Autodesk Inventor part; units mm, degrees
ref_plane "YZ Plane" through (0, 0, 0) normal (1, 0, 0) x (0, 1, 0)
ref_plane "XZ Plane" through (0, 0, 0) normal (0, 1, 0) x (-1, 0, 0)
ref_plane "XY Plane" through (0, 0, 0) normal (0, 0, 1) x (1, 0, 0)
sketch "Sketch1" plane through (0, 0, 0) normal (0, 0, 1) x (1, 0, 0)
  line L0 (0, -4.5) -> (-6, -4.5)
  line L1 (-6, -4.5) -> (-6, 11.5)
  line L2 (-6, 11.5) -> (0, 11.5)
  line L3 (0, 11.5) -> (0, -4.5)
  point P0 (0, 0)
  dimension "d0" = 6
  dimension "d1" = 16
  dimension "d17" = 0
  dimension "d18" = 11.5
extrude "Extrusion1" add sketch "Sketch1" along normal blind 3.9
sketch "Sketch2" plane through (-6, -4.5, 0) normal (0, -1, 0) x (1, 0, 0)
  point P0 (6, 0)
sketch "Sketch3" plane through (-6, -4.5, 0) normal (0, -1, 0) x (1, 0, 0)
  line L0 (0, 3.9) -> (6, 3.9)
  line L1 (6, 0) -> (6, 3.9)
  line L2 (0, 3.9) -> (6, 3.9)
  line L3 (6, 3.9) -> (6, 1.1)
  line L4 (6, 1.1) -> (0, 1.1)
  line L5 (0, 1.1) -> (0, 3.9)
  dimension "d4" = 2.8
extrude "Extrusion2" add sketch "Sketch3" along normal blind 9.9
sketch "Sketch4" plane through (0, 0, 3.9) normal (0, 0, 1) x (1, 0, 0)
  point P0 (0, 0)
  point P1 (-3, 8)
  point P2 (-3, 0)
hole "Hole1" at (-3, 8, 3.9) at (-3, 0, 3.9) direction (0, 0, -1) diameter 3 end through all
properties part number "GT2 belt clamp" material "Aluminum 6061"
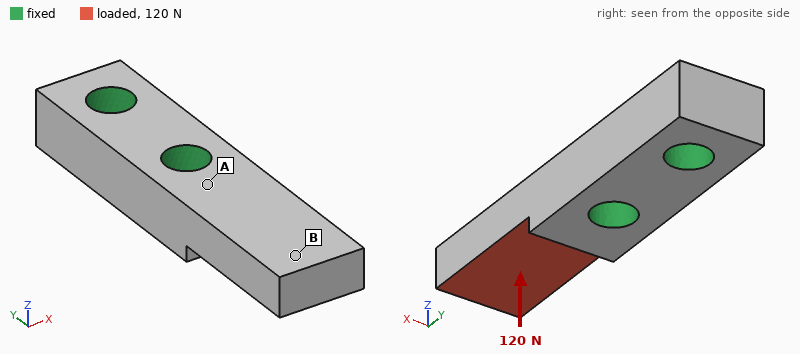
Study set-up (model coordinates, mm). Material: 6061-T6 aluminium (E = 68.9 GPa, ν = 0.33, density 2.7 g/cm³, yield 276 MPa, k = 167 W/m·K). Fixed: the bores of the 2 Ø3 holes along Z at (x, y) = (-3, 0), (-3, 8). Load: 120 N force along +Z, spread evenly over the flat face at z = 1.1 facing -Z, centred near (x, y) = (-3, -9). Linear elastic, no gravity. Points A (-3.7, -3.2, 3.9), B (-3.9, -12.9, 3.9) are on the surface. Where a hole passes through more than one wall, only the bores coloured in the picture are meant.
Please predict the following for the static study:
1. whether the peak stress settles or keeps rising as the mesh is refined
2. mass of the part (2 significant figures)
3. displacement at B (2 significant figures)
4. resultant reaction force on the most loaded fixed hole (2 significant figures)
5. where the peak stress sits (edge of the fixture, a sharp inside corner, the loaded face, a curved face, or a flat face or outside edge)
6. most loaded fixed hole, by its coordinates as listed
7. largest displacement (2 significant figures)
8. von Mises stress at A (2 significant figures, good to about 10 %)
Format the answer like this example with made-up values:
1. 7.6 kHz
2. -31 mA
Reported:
1. keeps rising
2. 1.3 g
3. 37 µm
4. 130 N
5. edge of the fixture
6. (-3, 0)
7. 43 µm
8. 66 MPa
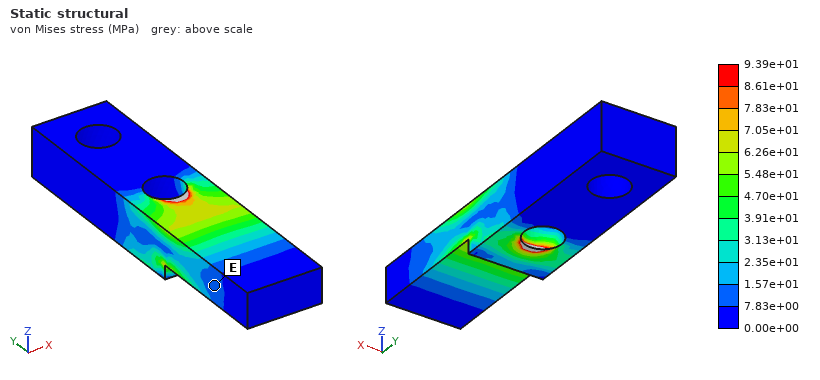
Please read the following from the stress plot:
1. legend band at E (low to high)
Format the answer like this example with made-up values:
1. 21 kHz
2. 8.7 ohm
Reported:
1. 7.83e+00 to 1.57e+01 MPa
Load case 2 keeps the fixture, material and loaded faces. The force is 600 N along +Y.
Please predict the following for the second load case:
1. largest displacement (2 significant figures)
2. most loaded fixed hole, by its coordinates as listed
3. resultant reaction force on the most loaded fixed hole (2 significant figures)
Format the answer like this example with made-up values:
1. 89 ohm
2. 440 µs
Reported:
1. 56 µm
2. (-3, 0)
3. 580 N
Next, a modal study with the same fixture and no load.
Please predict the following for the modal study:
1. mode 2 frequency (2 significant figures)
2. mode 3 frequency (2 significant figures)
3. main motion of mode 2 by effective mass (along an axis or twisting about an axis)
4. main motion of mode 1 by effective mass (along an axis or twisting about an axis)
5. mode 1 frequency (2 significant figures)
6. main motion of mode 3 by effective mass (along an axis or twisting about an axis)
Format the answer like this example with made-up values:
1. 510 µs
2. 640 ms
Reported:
1. 23 kHz
2. 48 kHz
3. along X
4. along Z
5. 15 kHz
6. twisting about Y
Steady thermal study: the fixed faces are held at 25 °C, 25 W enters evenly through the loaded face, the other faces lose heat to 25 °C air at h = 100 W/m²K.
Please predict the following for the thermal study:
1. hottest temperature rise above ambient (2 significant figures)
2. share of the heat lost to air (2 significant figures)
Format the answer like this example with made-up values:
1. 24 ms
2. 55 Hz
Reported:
1. 69 K
2. 3.2 %
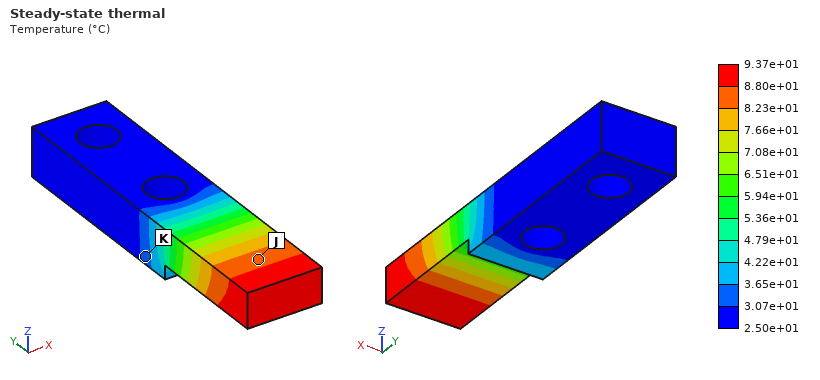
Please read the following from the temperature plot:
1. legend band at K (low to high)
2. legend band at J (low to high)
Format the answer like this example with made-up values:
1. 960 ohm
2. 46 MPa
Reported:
1. 3.07e+01 to 3.65e+01 °C
2. 8.23e+01 to 8.80e+01 °C
